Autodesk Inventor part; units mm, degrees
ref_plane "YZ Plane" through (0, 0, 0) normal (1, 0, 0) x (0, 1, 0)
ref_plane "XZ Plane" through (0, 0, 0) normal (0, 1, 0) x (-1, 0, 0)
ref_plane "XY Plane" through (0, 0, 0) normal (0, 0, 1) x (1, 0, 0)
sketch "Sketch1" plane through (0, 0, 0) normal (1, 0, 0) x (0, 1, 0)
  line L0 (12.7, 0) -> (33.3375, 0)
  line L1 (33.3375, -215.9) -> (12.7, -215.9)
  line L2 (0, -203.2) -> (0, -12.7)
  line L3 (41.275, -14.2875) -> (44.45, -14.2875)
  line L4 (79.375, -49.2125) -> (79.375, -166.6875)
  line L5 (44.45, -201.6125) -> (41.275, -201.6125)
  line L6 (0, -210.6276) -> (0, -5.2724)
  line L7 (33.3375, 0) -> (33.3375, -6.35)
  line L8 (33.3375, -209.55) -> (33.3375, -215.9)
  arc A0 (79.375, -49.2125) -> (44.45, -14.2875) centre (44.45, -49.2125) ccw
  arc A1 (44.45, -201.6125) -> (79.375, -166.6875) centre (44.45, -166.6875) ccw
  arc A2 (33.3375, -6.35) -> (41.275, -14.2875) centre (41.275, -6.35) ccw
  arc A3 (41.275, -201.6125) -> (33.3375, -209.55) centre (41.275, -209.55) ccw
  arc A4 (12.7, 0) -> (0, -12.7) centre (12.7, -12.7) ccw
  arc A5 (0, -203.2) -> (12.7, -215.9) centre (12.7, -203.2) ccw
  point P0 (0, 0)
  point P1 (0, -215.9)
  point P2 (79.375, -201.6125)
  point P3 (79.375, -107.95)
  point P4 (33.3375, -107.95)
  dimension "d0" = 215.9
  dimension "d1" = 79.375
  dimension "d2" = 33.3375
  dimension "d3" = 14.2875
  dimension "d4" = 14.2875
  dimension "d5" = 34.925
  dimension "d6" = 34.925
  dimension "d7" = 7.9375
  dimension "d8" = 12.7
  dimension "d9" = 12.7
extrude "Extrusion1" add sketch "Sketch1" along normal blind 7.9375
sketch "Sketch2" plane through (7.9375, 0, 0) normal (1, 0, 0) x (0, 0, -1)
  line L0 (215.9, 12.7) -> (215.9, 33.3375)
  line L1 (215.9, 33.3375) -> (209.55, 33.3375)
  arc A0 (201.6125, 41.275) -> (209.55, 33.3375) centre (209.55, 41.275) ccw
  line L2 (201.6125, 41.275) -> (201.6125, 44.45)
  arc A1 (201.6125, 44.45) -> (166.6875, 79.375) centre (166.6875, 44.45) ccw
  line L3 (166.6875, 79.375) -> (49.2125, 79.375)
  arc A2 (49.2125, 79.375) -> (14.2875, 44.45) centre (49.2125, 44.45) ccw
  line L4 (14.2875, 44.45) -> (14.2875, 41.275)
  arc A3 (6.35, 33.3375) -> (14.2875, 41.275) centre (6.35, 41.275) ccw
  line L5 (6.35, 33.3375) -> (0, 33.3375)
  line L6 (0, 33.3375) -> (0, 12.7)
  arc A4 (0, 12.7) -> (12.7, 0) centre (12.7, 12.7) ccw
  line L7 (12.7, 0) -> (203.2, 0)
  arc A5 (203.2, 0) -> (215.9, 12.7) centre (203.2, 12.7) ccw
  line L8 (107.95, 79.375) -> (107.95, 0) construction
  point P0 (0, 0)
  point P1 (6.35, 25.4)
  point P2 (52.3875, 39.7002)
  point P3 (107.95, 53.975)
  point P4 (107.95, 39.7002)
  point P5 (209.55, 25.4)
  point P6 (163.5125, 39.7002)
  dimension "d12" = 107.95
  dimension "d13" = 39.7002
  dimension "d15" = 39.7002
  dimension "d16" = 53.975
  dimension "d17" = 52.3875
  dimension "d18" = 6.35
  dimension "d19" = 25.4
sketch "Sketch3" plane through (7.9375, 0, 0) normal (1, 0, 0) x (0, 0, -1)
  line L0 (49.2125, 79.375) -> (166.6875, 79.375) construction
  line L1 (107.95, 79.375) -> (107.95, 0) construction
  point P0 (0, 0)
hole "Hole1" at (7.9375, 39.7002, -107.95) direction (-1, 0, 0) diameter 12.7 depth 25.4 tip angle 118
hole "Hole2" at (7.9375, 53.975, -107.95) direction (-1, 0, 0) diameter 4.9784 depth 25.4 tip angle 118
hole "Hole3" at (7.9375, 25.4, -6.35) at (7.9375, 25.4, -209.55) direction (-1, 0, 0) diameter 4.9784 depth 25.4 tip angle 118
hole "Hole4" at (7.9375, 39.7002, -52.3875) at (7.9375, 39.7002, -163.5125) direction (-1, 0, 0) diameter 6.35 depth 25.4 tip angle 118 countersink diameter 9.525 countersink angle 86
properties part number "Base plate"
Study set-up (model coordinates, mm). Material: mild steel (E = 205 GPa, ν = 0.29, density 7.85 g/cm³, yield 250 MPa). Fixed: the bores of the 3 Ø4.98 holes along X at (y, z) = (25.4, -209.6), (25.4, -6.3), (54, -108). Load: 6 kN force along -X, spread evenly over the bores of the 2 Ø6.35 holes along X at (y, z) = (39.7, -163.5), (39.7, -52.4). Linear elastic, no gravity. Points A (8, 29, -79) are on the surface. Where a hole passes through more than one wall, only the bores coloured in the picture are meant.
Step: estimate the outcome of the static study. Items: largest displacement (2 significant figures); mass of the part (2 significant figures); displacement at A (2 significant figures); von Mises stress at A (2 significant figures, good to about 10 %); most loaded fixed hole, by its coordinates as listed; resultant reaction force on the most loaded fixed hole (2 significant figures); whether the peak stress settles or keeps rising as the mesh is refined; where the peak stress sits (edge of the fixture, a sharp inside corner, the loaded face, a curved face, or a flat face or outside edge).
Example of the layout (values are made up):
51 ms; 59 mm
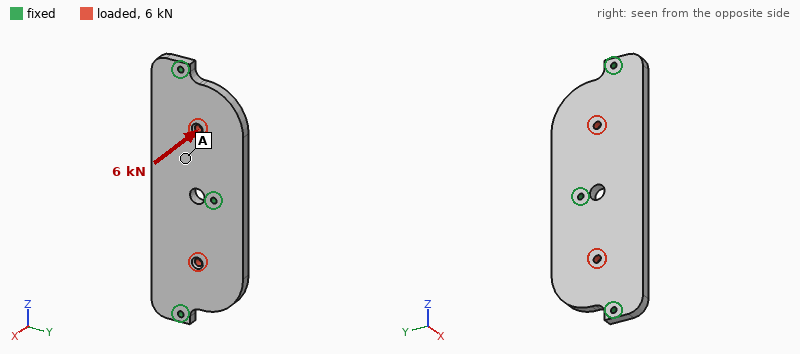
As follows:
52 µm; 930 g; 34 µm; 27 MPa; (54, -108); 3.0 kN; keeps rising; edge of the fixture
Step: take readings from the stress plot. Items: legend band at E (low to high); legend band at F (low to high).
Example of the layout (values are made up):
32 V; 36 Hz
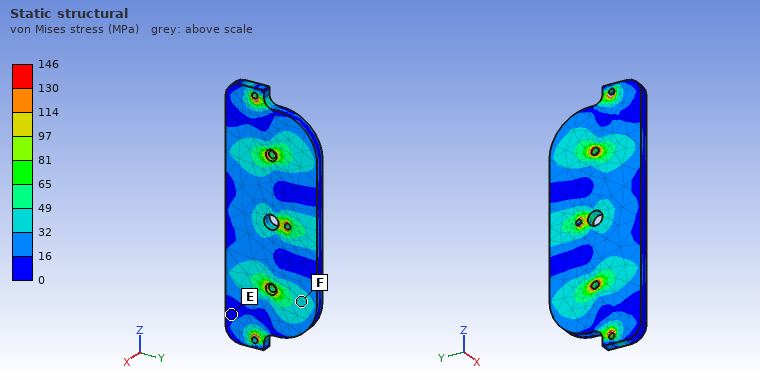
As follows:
0 to 16 MPa; 32 to 49 MPa
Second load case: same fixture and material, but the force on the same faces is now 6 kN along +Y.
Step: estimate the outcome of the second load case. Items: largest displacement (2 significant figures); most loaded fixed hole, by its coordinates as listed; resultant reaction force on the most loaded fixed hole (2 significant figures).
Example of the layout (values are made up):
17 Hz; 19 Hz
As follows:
5.3 µm; (54, -108); 3.4 kN
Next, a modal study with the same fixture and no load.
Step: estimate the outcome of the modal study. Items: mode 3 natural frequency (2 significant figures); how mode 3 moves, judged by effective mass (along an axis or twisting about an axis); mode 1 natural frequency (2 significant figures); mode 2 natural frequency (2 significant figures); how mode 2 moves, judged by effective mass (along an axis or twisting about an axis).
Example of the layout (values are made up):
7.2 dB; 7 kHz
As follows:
2500 Hz; along X; 1700 Hz; 2200 Hz; twisting about Y
